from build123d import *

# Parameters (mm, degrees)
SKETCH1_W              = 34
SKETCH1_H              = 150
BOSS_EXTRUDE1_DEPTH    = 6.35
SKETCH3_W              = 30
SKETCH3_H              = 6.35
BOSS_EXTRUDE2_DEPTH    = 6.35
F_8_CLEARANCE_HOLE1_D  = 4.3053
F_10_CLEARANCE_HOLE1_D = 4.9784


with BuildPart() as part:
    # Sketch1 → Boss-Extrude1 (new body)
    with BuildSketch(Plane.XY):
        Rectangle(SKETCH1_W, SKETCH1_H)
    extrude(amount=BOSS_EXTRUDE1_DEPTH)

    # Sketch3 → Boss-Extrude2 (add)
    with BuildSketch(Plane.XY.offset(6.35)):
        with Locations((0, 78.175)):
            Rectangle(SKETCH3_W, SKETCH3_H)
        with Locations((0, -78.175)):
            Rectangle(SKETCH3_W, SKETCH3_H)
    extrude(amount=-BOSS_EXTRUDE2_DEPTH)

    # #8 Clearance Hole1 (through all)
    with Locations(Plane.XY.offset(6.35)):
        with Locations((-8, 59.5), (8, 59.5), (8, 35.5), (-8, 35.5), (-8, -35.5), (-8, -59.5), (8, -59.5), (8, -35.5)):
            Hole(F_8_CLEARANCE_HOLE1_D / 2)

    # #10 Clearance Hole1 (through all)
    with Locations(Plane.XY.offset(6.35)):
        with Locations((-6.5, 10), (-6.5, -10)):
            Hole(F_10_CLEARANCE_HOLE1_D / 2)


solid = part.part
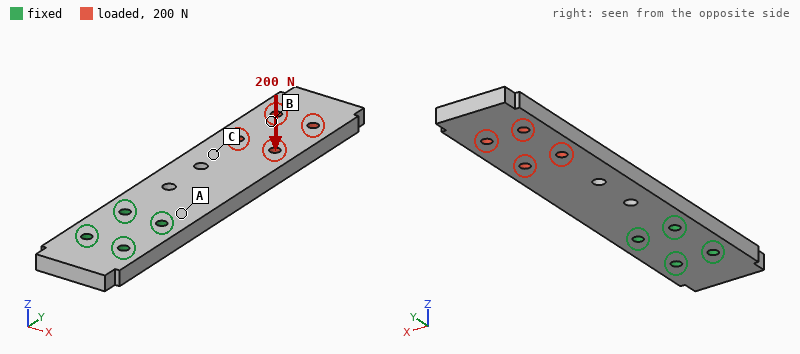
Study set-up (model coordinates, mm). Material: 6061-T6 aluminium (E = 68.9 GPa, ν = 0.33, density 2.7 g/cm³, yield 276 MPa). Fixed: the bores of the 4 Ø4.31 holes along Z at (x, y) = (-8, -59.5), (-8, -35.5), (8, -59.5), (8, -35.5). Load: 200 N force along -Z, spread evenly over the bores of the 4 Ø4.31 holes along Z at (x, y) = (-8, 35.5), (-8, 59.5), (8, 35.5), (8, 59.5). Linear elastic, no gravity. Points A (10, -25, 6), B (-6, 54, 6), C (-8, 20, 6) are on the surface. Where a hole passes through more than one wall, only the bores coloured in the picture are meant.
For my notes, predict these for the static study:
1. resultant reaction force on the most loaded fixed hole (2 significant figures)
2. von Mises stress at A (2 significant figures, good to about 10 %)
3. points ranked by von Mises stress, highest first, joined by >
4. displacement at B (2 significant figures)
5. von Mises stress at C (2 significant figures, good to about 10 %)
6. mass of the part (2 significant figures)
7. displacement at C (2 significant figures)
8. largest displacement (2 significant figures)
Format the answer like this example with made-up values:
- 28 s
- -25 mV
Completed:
- 170 N
- 62 MPa
- A > C > B
- 0.86 mm
- 23 MPa
- 91 g
- 0.40 mm
- 1.3 mm
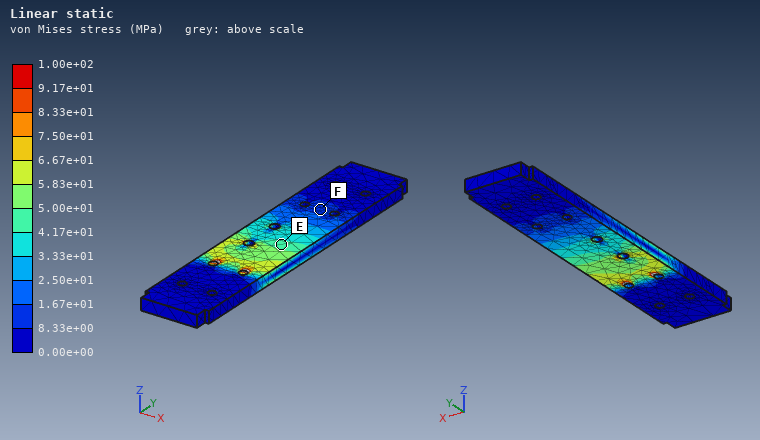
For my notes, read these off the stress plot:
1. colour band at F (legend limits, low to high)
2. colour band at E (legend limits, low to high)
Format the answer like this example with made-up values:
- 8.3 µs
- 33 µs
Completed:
- 8.33e+00 to 1.67e+01 MPa
- 4.17e+01 to 5.00e+01 MPa
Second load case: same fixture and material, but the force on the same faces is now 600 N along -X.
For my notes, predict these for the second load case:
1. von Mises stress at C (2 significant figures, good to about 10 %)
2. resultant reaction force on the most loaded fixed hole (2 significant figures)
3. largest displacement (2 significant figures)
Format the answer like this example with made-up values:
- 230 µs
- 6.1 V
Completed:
- 9.1 MPa
- 2.1 kN
- 0.16 mm
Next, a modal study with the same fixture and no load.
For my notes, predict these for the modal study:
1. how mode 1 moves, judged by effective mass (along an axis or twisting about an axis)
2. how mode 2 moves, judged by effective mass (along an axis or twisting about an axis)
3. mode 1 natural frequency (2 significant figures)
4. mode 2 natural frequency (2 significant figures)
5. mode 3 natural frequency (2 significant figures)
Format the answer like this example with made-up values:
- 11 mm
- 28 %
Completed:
- along Z
- along X
- 390 Hz
- 1800 Hz
- 2400 Hz
